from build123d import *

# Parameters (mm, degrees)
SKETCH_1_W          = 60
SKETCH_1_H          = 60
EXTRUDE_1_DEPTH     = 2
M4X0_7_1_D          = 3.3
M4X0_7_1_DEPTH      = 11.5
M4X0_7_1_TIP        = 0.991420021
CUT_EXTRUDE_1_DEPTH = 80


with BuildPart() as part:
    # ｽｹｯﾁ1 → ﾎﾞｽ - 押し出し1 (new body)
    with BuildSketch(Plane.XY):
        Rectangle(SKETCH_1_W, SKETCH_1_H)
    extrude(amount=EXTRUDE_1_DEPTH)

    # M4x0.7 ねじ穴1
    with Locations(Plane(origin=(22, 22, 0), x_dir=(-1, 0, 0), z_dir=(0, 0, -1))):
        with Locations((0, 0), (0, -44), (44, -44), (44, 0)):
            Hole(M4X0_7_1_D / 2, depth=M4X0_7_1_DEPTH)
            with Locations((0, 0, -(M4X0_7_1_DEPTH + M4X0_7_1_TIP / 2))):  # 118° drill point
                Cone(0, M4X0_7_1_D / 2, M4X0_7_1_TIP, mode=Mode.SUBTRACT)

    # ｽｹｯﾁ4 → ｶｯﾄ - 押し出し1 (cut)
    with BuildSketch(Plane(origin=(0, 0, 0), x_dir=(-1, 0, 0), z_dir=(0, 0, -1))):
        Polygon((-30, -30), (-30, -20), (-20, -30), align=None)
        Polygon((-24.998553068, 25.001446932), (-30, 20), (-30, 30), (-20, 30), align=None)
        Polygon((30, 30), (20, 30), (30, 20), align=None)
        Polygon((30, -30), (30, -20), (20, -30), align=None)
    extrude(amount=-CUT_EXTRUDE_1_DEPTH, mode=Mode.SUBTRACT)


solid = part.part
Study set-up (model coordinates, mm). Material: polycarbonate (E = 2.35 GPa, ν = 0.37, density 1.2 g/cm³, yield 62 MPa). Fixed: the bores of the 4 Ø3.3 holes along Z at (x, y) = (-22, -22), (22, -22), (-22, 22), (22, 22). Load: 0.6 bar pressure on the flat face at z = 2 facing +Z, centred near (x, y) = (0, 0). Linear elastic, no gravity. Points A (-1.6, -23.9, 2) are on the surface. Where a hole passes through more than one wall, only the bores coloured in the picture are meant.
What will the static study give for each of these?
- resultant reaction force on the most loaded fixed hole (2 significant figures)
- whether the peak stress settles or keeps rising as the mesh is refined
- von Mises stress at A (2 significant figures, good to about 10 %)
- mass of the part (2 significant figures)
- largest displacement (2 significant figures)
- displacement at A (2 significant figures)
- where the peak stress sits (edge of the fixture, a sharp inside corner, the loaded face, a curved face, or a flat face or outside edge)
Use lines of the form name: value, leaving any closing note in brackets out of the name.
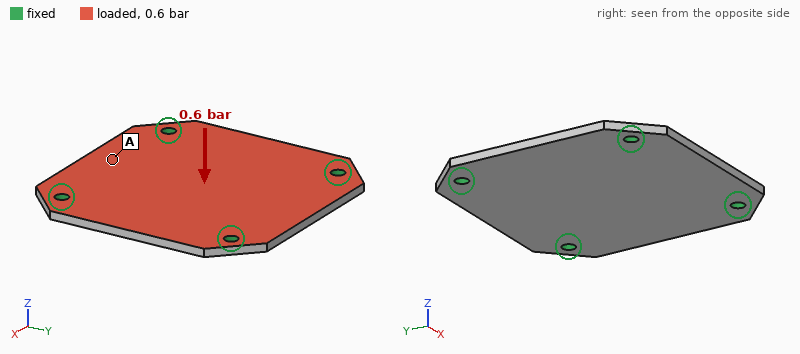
resultant reaction force on the most loaded fixed hole: 50 N
whether the peak stress settles or keeps rising as the mesh is refined: keeps rising
von Mises stress at A: 7.9 MPa
mass of the part: 8.1 g
largest displacement: 0.81 mm
displacement at A: 0.42 mm
where the peak stress sits: edge of the fixture
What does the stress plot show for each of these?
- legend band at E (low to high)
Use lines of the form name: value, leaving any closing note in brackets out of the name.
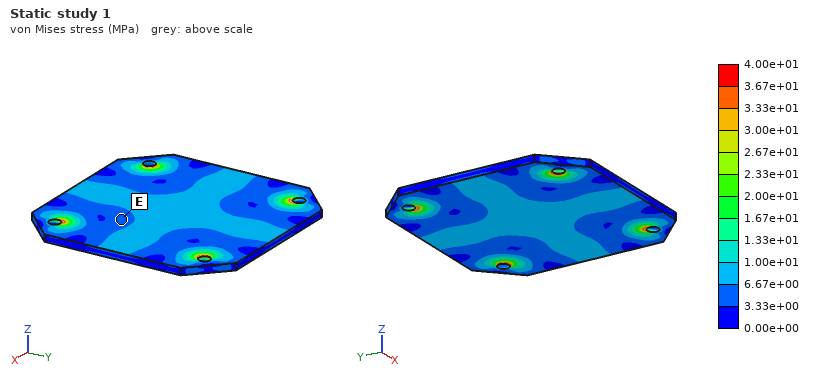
legend band at E: 3.33e+00 to 6.67e+00 MPa
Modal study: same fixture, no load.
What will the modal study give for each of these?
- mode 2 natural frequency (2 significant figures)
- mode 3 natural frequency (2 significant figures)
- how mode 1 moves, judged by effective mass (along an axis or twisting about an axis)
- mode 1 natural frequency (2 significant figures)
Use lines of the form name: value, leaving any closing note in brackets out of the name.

mode 2 natural frequency: 1600 Hz
mode 3 natural frequency: 1600 Hz
how mode 1 moves, judged by effective mass: along Z
mode 1 natural frequency: 1100 Hz
